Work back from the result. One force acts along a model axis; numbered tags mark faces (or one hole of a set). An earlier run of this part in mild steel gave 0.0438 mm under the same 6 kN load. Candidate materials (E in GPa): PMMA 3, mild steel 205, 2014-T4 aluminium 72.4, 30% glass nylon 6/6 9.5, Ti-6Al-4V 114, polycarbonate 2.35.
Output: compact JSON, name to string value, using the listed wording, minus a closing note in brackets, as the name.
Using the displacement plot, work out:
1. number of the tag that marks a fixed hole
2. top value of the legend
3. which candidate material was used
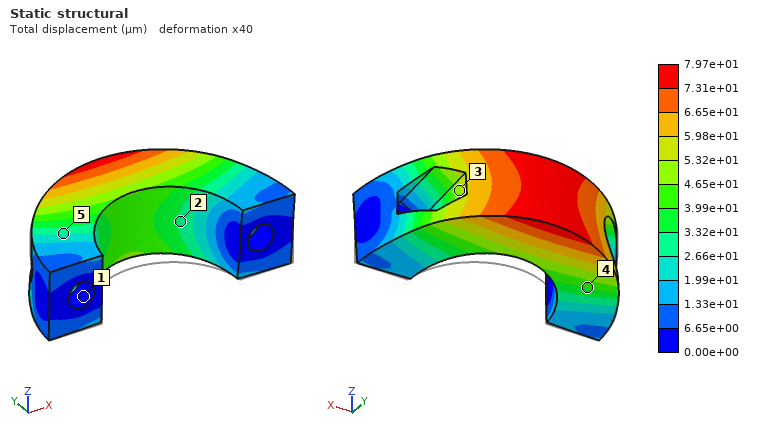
{"number of the tag that marks a fixed hole": "1", "top value of the legend": "7.97e+01 µm", "which candidate material was used": "Ti-6Al-4V"}
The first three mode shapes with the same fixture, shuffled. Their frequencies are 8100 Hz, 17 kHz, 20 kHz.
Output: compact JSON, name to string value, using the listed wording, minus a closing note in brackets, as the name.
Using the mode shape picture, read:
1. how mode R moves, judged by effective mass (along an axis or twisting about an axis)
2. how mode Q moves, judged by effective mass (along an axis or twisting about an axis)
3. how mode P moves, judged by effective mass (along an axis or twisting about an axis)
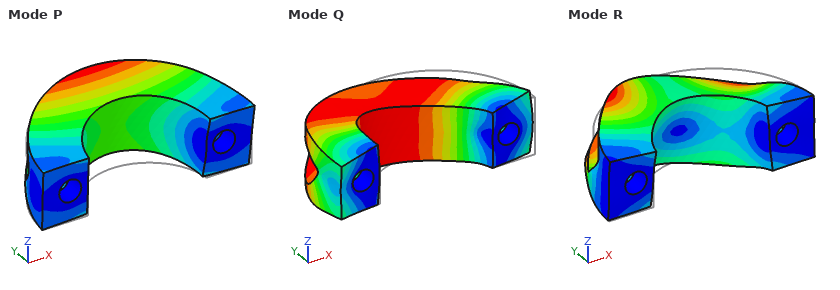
{"how mode R moves, judged by effective mass": "twisting about Y", "how mode Q moves, judged by effective mass": "along X", "how mode P moves, judged by effective mass": "along Z"}
